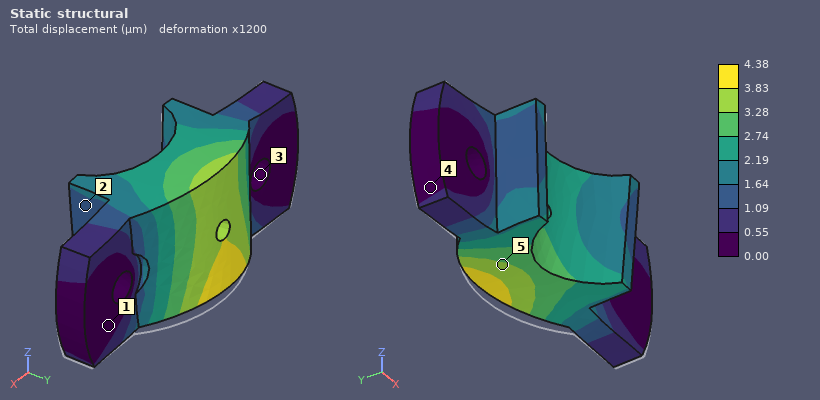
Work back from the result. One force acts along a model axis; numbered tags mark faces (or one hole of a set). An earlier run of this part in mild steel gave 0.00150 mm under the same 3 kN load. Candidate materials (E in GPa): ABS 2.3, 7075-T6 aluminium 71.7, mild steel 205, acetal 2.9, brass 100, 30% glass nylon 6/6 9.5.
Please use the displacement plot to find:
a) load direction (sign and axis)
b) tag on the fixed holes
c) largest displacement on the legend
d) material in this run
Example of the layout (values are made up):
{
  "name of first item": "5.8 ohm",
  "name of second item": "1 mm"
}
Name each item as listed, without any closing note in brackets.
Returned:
{
  "load direction": "+Z",
  "tag on the fixed holes": "3",
  "largest displacement on the legend": "4.38 µm",
  "material in this run": "7075-T6 aluminium"
}
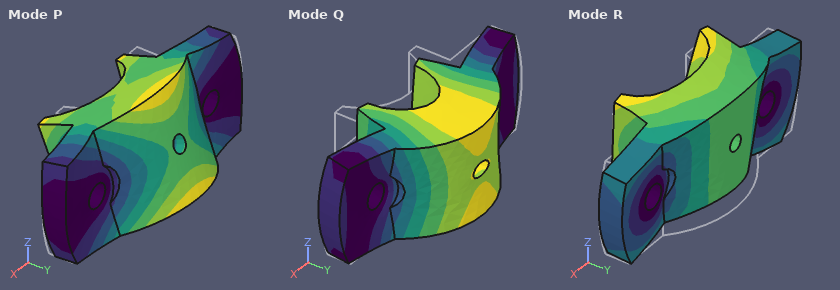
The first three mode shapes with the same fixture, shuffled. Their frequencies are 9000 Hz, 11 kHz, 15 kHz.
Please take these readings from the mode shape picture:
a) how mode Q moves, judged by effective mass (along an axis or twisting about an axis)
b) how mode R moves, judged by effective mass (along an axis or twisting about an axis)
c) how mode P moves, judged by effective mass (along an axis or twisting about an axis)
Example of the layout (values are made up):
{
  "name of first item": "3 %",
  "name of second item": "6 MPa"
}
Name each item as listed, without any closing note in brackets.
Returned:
{
  "how mode Q moves, judged by effective mass": "along Y",
  "how mode R moves, judged by effective mass": "along Z",
  "how mode P moves, judged by effective mass": "twisting about X"
}
